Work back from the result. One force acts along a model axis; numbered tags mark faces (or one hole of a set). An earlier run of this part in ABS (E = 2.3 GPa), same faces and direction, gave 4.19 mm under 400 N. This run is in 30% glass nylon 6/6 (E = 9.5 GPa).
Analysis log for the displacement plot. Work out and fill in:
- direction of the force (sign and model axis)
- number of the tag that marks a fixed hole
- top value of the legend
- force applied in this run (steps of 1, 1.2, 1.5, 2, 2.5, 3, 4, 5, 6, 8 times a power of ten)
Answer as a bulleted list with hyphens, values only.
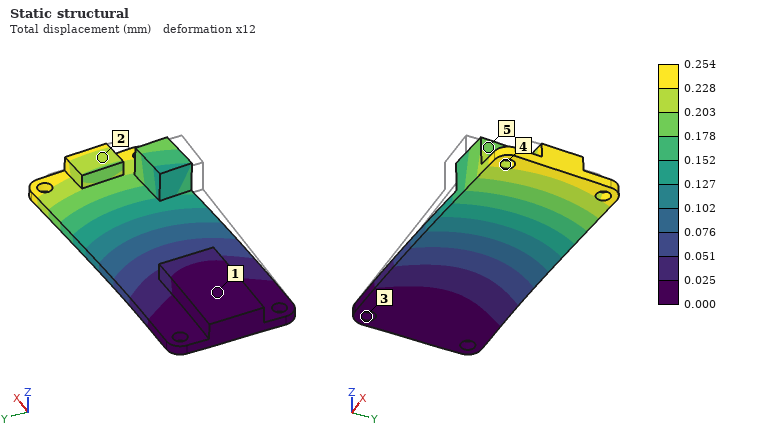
- +Y
- 3
- 0.254 mm
- 100 N
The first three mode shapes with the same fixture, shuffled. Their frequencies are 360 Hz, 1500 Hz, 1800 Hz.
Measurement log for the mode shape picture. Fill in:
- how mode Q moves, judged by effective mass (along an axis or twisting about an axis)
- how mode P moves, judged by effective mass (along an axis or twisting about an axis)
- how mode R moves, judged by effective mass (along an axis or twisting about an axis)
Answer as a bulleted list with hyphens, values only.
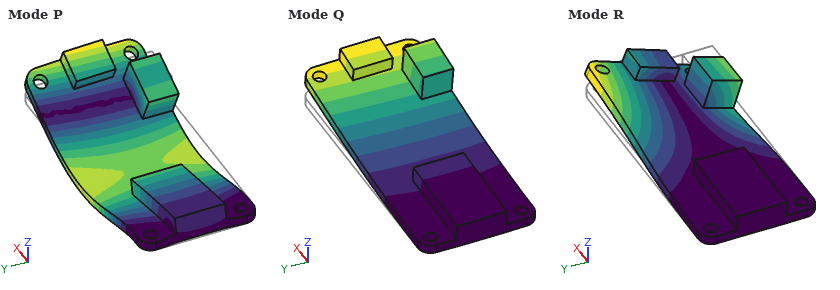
- along Z
- along Z
- twisting about X
